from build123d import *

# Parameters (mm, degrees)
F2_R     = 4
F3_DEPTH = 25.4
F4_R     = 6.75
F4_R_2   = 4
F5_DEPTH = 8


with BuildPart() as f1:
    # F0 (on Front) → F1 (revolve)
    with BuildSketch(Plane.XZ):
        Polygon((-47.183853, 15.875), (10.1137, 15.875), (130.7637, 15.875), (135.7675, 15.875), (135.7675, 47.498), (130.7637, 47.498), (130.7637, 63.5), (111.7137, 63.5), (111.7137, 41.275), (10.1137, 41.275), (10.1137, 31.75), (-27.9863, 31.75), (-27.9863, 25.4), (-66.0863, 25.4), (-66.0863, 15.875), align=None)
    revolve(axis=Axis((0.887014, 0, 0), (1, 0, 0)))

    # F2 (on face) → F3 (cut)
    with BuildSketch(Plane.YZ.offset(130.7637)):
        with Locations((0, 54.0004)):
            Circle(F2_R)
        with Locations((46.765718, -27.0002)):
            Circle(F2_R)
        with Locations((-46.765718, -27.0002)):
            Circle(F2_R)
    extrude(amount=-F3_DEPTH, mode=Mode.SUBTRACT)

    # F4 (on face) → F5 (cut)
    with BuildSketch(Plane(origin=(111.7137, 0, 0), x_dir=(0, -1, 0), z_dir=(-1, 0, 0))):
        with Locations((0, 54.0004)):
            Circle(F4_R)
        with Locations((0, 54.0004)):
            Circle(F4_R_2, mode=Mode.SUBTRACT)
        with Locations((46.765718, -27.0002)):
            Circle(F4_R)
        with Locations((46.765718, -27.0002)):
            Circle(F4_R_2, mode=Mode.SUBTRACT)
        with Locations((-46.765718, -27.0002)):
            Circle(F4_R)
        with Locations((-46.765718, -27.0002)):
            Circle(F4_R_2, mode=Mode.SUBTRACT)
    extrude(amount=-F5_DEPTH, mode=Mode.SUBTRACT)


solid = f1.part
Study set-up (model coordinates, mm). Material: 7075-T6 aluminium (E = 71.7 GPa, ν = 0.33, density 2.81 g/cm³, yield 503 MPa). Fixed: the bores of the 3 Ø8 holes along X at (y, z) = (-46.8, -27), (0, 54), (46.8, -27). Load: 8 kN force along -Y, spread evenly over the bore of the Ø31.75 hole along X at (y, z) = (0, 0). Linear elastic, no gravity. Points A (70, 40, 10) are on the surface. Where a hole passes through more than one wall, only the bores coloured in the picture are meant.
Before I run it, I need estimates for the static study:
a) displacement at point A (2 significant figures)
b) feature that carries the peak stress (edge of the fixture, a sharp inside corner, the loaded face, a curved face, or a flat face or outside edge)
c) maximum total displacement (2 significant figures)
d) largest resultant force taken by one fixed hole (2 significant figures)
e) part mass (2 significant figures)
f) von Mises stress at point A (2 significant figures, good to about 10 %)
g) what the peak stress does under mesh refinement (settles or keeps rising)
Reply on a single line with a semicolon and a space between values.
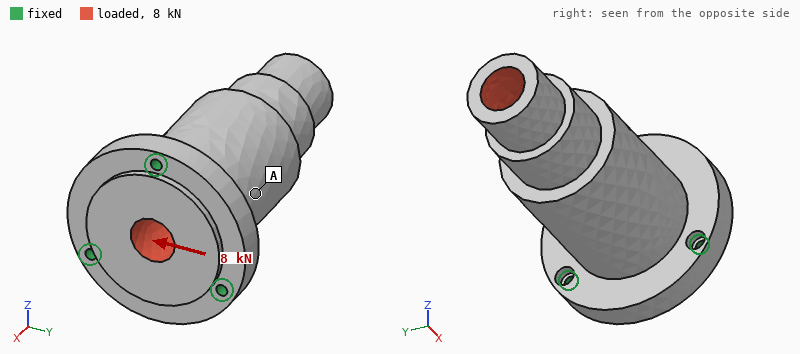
0.035 mm; edge of the fixture; 0.12 mm; 8.6 kN; 2.4 kg; 6.2 MPa; keeps rising
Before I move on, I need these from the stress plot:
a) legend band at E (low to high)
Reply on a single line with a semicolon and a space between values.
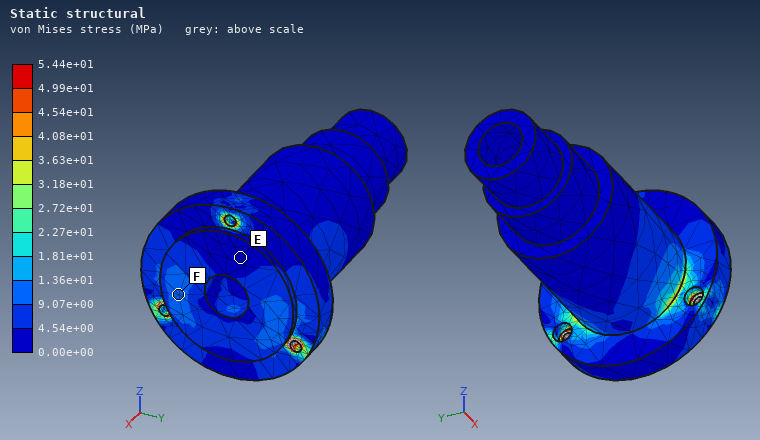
0.00e+00 to 4.54e+00 MPa
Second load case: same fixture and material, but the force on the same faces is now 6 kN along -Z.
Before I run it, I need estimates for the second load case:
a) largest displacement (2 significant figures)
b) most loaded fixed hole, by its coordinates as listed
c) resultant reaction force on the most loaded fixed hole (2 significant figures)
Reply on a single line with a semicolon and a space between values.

90 µm; (0, 54); 7.5 kN
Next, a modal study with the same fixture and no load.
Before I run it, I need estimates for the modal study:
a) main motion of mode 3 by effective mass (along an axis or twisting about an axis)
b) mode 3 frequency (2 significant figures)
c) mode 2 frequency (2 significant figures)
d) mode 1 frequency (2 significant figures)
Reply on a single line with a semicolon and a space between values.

along X; 3700 Hz; 1400 Hz; 1400 Hz
